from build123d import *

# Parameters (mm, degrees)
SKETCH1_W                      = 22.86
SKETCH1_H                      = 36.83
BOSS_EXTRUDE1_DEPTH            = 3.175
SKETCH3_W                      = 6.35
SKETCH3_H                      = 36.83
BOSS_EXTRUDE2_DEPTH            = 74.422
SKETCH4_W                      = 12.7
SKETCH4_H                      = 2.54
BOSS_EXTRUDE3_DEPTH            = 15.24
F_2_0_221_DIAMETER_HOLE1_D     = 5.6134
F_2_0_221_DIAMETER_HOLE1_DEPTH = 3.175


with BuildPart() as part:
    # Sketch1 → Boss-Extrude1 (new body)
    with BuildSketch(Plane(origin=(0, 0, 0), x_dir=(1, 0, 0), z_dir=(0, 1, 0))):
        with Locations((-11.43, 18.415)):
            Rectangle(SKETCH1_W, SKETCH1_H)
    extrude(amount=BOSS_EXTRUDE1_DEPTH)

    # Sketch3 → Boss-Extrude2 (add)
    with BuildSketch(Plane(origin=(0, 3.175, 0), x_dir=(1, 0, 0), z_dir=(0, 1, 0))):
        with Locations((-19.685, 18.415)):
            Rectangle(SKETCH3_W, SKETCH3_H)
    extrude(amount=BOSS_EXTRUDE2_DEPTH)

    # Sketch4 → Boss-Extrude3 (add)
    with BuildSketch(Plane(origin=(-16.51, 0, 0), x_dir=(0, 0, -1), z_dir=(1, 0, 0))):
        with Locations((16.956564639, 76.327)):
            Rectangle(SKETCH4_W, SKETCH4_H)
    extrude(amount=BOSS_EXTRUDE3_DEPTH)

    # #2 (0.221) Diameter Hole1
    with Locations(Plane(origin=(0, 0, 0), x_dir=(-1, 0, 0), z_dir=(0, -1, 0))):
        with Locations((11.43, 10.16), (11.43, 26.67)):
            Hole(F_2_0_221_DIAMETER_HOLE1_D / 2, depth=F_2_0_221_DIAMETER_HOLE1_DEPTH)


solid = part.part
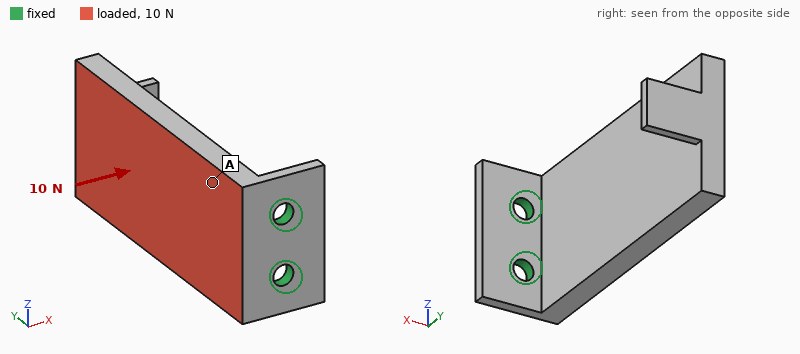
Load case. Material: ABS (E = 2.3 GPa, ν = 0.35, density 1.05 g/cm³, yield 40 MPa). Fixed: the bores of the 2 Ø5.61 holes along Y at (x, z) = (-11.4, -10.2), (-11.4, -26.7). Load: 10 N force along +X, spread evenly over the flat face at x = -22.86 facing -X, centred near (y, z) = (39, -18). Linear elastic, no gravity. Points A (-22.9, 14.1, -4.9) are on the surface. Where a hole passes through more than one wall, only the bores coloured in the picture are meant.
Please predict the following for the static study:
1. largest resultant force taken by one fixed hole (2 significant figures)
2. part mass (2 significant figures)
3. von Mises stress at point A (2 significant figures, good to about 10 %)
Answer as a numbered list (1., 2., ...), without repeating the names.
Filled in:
1. 5.5 N
2. 21 g
3. 1.0 MPa
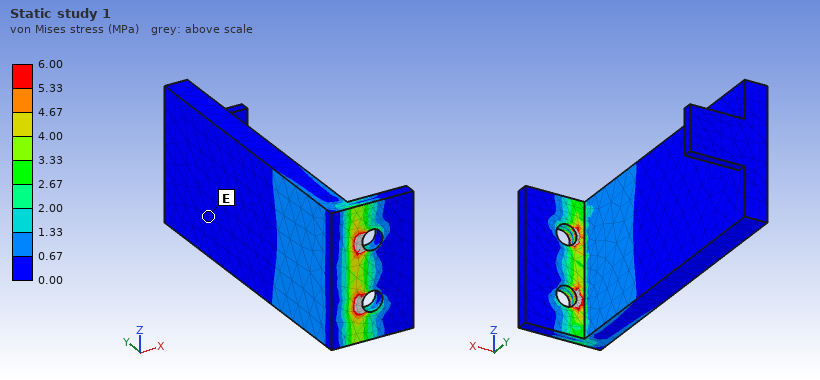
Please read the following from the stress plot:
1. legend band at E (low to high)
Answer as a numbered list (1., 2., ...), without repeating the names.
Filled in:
1. 0.00 to 0.67 MPa
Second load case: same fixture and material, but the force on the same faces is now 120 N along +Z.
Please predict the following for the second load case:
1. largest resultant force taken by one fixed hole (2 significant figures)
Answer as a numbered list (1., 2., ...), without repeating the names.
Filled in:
1. 240 N
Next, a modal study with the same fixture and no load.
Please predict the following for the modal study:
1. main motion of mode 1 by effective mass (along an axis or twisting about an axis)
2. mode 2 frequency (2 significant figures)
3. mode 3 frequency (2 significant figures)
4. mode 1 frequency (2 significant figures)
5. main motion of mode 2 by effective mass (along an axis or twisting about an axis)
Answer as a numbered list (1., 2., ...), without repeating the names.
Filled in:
1. along X
2. 490 Hz
3. 980 Hz
4. 140 Hz
5. along Z
